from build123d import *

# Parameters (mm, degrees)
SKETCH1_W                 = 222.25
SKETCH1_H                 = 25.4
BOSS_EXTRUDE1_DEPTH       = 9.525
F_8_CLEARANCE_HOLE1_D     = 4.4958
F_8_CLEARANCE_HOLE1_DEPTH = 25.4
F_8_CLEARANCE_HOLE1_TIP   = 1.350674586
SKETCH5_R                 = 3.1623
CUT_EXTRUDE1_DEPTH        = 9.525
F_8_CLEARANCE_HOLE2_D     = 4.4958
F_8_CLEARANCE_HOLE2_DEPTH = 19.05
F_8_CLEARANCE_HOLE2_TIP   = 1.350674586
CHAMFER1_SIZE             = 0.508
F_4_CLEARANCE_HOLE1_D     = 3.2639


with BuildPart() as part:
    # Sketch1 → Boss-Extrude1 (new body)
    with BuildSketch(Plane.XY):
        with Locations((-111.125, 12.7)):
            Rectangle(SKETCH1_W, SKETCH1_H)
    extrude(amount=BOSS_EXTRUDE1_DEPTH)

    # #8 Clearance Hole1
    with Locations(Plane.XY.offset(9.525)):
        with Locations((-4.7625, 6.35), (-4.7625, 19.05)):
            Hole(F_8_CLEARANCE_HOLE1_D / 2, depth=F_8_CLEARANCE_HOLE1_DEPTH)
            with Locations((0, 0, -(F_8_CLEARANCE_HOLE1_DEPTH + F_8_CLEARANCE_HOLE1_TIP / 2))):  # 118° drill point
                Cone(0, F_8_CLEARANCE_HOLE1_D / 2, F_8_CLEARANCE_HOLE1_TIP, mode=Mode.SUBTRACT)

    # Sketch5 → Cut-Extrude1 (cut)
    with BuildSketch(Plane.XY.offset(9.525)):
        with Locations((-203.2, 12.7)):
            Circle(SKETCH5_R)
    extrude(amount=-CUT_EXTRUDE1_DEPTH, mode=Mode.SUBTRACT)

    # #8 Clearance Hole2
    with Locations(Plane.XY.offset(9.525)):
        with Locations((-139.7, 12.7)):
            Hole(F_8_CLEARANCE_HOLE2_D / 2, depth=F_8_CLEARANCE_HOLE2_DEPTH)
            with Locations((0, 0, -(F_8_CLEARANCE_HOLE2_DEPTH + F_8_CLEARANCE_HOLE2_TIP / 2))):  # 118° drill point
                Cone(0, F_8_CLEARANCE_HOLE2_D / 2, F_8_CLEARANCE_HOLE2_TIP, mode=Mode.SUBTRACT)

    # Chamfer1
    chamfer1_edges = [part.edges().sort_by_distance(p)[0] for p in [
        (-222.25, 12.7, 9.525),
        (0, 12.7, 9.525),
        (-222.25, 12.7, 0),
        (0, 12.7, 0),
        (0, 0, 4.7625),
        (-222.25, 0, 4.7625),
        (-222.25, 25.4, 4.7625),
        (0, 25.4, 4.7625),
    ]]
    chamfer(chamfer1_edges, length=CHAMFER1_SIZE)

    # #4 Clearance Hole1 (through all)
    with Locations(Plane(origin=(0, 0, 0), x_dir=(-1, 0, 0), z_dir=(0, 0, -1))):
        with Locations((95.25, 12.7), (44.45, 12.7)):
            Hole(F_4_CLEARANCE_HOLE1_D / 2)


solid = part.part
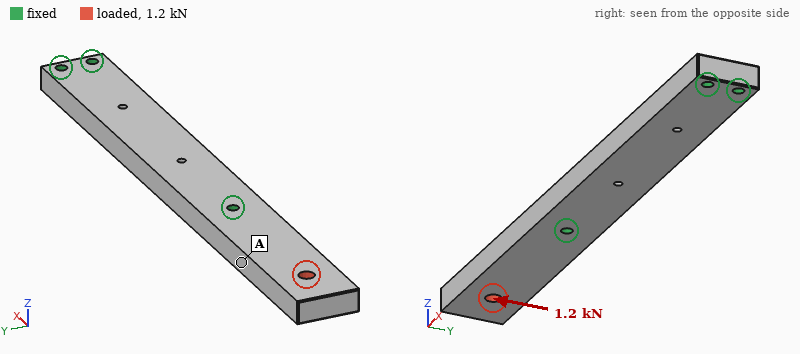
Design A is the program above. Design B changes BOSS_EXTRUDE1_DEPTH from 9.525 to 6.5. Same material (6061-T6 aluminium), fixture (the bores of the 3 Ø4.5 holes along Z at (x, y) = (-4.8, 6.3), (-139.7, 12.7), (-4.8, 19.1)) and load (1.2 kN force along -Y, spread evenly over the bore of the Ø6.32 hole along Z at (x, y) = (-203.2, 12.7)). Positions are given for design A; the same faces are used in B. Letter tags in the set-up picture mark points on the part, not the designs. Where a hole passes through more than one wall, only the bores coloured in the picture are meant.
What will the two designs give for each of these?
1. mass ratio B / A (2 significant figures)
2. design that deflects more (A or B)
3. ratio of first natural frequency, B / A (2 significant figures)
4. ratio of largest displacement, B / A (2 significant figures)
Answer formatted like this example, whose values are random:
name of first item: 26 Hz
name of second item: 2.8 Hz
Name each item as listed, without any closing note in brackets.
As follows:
mass ratio B / A: 0.68
design that deflects more: B
ratio of first natural frequency, B / A: 0.70
ratio of largest displacement, B / A: 1.5
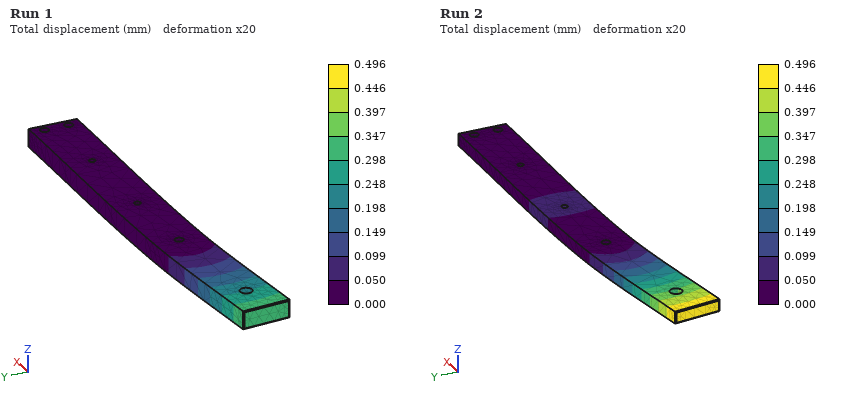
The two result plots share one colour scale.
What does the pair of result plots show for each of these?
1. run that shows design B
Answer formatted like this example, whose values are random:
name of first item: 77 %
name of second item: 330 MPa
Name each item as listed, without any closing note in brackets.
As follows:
run that shows design B: Run 2
